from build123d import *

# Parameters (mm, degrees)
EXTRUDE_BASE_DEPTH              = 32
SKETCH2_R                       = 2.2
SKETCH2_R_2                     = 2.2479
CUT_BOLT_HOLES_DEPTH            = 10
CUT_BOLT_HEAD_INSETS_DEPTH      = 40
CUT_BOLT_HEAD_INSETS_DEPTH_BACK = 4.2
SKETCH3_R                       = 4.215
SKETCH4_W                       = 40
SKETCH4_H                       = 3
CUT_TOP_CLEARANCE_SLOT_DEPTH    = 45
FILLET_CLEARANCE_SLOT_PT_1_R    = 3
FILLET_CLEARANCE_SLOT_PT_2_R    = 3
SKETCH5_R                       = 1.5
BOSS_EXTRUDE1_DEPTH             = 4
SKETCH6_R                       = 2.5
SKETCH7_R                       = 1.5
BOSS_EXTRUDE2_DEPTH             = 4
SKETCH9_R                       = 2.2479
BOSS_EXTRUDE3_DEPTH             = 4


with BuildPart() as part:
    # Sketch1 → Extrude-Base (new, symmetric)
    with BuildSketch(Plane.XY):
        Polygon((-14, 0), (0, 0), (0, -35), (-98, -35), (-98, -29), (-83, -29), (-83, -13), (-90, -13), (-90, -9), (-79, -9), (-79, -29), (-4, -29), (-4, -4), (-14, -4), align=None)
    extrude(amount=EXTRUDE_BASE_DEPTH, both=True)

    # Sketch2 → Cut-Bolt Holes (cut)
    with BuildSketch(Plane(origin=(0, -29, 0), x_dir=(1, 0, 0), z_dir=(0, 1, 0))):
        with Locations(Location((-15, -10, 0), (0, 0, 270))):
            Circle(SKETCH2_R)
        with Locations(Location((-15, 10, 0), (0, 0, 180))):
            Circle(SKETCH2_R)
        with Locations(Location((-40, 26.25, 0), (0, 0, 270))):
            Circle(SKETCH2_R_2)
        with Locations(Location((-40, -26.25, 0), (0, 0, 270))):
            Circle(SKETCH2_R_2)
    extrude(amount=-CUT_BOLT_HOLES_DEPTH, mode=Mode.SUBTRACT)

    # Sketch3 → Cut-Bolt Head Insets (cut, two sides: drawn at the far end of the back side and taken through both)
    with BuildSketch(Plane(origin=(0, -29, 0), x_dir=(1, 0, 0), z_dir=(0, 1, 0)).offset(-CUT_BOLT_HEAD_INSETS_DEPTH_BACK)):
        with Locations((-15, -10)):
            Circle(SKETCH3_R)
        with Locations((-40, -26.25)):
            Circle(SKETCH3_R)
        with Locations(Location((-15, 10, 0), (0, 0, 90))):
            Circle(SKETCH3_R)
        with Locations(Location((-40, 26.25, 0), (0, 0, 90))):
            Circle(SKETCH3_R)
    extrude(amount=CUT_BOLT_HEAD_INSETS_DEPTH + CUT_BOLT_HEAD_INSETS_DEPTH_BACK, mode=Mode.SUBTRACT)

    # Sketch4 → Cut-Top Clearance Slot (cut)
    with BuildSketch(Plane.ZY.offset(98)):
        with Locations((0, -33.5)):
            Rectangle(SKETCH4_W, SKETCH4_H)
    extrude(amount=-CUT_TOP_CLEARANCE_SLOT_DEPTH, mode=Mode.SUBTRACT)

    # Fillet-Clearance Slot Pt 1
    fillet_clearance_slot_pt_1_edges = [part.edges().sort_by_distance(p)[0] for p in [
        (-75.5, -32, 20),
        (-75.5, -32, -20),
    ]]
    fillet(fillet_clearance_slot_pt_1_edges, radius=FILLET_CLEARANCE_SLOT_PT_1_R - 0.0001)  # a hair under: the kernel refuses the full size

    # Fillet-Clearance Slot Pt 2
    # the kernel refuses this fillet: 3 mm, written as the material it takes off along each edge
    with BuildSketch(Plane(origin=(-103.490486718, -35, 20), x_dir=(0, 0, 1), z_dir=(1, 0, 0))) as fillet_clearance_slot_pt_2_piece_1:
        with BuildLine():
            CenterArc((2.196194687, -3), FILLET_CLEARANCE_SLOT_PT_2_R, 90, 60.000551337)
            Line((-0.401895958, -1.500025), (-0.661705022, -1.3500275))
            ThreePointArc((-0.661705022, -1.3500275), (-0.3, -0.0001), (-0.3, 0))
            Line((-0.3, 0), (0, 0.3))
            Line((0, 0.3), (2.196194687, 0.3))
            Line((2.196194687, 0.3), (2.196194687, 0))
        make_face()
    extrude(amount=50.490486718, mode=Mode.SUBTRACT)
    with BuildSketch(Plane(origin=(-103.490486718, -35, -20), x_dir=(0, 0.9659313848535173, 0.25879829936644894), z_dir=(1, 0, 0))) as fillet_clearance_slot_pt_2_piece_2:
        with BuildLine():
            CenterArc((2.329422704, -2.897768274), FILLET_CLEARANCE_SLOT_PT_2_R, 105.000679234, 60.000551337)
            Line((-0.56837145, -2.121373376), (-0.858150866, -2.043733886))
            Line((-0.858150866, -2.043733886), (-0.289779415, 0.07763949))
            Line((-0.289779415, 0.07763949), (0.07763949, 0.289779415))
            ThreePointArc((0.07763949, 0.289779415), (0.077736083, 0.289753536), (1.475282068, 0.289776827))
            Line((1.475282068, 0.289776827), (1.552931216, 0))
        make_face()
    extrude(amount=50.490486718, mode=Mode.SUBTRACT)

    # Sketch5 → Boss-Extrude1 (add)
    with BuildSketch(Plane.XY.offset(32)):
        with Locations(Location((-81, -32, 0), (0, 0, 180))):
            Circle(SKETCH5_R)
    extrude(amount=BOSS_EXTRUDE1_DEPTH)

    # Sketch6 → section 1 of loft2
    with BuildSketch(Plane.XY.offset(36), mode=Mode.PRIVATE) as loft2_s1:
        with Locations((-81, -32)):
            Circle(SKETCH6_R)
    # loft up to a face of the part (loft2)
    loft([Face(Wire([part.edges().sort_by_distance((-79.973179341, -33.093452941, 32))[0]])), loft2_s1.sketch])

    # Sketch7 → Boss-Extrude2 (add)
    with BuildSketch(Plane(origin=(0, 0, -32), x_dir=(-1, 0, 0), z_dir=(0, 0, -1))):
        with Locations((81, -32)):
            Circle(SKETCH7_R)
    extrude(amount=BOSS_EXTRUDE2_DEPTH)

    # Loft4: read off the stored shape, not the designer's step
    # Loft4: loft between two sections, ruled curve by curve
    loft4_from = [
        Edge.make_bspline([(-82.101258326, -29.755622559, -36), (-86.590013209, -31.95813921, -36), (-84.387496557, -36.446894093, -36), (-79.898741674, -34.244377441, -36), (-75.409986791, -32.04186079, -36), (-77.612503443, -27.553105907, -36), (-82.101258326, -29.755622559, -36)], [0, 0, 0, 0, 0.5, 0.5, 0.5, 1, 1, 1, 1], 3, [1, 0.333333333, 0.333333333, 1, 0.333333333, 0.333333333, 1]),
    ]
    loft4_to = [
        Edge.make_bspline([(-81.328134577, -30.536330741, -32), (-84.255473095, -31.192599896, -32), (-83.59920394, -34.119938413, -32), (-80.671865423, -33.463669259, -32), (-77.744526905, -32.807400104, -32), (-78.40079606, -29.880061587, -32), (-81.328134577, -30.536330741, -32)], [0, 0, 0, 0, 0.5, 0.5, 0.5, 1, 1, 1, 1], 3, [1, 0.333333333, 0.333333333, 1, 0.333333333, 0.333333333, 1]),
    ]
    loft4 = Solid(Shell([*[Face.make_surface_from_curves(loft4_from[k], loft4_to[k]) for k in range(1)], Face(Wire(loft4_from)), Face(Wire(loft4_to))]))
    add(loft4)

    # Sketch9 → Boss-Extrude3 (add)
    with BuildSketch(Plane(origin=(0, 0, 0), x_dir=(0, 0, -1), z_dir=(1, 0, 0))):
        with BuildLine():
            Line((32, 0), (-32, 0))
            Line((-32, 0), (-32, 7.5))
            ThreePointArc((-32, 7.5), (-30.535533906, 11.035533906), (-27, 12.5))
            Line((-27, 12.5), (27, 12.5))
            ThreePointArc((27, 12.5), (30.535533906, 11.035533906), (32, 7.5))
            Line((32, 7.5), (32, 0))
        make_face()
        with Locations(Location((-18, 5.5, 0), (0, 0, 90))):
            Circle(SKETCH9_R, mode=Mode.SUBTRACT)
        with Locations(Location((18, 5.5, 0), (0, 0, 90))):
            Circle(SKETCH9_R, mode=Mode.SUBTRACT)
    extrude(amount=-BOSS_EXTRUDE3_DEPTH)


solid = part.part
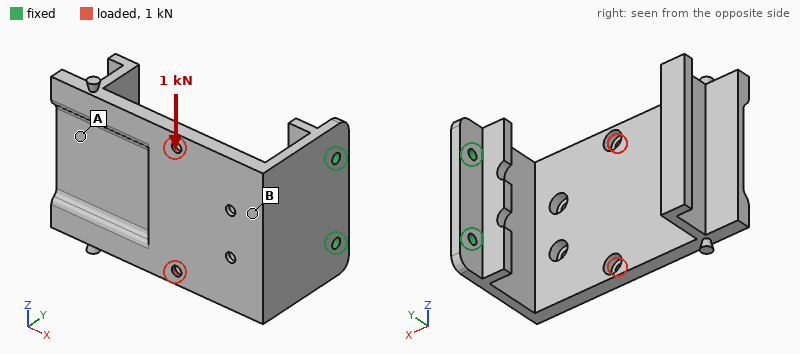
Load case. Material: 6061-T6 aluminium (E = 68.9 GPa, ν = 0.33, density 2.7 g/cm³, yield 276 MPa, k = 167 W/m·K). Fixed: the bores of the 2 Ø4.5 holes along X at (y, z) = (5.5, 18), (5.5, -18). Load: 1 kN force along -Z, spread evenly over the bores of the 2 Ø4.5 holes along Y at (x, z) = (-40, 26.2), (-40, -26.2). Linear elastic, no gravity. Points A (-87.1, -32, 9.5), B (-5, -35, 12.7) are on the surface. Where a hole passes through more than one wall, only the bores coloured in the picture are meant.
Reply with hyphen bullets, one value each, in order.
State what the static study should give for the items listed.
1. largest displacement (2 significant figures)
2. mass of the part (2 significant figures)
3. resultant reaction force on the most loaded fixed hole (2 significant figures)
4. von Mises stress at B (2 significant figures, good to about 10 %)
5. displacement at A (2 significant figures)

- 1.5 mm
- 140 g
- 1.5 kN
- 45 MPa
- 1.3 mm
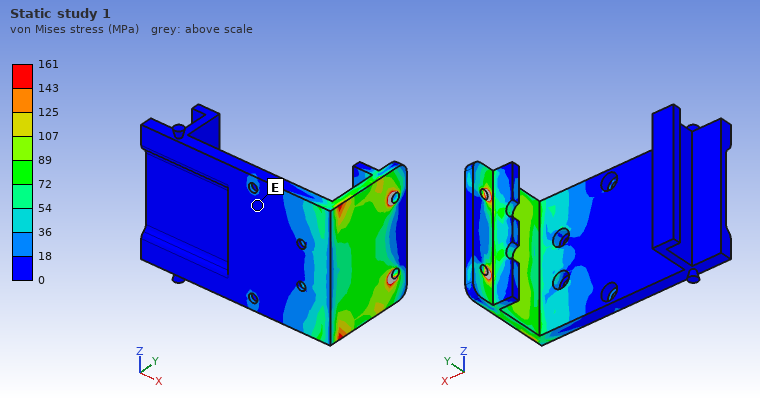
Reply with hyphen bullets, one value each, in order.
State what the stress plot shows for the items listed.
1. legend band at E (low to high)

- 0 to 18 MPa
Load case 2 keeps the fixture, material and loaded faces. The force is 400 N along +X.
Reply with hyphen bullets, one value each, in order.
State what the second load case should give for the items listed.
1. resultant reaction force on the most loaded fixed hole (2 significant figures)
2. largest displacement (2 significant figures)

- 210 N
- 1.3 mm
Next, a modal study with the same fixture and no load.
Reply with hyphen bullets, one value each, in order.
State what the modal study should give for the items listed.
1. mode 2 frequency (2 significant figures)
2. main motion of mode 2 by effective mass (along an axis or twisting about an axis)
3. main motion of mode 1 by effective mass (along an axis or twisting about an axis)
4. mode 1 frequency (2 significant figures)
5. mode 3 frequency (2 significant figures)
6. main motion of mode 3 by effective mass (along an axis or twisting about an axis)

- 400 Hz
- along Z
- along Y
- 200 Hz
- 860 Hz
- along X
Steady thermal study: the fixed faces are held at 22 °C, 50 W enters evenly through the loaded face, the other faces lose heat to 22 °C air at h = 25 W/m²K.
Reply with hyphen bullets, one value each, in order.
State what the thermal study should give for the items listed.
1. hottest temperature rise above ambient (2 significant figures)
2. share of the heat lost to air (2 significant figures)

- 66 K
- 42 %
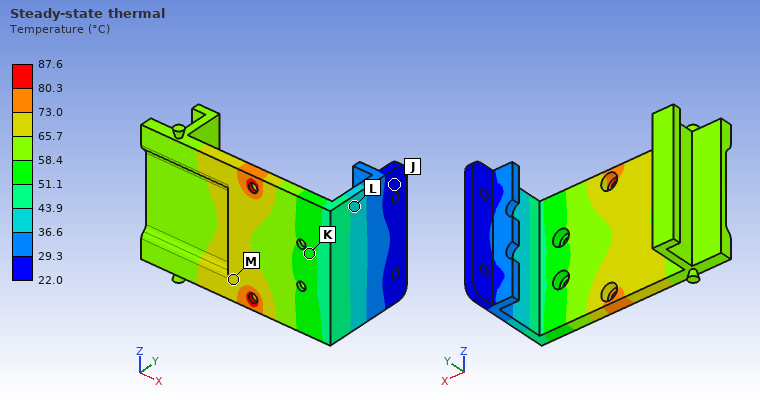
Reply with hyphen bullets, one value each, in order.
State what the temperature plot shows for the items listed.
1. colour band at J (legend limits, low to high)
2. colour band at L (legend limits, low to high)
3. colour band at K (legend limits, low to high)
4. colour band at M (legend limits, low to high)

- 22.0 to 29.3 °C
- 36.6 to 43.9 °C
- 51.1 to 58.4 °C
- 65.7 to 73.0 °C
